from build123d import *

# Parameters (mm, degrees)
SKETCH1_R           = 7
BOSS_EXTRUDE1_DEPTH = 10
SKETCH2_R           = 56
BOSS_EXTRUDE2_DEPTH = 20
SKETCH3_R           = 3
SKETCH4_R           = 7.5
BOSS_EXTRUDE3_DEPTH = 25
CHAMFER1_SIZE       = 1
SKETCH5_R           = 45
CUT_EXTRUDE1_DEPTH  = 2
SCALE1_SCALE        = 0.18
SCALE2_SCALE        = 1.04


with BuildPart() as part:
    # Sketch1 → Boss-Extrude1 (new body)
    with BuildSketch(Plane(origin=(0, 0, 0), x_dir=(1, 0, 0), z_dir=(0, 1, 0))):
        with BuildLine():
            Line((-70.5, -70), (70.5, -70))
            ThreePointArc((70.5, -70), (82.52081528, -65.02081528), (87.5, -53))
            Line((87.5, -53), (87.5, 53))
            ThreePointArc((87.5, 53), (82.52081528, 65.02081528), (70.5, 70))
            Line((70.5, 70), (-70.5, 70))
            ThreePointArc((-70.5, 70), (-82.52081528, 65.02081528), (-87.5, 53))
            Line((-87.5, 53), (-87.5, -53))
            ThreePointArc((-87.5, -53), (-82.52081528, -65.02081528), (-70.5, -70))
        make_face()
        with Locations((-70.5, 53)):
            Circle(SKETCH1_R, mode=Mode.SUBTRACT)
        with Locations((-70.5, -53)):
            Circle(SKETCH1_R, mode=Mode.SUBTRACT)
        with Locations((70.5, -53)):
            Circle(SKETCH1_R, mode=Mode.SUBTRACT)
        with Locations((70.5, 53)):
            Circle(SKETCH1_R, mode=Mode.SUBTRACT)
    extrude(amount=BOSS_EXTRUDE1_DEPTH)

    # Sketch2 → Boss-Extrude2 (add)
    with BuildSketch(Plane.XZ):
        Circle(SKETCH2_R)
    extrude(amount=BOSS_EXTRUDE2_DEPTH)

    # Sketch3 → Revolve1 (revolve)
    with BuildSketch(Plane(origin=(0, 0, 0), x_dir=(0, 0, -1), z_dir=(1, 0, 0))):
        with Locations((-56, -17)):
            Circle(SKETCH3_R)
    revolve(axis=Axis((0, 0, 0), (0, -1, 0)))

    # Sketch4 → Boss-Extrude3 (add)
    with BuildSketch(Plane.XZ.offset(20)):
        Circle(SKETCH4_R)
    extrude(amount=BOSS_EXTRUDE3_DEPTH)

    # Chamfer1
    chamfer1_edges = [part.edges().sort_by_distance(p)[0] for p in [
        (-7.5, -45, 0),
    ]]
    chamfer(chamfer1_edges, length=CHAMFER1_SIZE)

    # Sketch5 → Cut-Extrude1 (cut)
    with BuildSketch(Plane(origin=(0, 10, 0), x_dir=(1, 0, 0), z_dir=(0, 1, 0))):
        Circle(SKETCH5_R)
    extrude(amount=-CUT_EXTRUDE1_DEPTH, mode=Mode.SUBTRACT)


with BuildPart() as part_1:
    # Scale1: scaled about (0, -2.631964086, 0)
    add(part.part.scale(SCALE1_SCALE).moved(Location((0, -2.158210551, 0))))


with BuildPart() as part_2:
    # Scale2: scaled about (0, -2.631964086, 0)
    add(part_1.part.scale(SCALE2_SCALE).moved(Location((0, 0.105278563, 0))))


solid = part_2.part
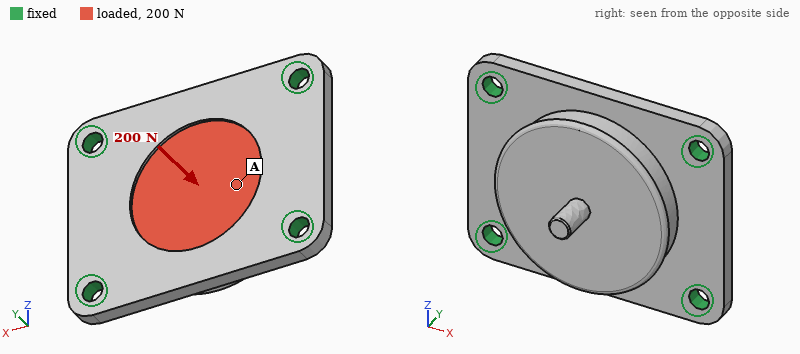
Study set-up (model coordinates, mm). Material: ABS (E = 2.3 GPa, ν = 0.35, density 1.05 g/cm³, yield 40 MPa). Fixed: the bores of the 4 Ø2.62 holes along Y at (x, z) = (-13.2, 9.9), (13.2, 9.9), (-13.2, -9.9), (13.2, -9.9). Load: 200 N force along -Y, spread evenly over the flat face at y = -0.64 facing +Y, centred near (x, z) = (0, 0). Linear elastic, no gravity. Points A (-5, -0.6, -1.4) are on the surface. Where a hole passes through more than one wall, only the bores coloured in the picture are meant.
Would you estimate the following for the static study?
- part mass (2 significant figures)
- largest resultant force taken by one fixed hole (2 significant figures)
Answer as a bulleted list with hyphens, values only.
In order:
- 3.0 g
- 61 N
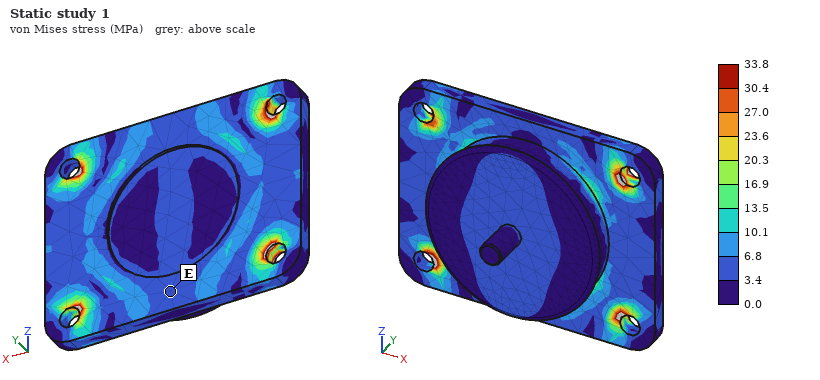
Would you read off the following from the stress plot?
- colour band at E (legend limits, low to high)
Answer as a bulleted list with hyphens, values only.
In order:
- 3.4 to 6.8 MPa
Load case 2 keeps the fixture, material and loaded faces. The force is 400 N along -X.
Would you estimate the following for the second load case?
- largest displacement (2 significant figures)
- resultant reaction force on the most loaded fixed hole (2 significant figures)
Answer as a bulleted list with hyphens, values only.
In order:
- 40 µm
- 100 N
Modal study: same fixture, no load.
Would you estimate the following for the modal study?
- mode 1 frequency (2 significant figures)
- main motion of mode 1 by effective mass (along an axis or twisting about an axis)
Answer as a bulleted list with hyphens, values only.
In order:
- 4000 Hz
- along Y
